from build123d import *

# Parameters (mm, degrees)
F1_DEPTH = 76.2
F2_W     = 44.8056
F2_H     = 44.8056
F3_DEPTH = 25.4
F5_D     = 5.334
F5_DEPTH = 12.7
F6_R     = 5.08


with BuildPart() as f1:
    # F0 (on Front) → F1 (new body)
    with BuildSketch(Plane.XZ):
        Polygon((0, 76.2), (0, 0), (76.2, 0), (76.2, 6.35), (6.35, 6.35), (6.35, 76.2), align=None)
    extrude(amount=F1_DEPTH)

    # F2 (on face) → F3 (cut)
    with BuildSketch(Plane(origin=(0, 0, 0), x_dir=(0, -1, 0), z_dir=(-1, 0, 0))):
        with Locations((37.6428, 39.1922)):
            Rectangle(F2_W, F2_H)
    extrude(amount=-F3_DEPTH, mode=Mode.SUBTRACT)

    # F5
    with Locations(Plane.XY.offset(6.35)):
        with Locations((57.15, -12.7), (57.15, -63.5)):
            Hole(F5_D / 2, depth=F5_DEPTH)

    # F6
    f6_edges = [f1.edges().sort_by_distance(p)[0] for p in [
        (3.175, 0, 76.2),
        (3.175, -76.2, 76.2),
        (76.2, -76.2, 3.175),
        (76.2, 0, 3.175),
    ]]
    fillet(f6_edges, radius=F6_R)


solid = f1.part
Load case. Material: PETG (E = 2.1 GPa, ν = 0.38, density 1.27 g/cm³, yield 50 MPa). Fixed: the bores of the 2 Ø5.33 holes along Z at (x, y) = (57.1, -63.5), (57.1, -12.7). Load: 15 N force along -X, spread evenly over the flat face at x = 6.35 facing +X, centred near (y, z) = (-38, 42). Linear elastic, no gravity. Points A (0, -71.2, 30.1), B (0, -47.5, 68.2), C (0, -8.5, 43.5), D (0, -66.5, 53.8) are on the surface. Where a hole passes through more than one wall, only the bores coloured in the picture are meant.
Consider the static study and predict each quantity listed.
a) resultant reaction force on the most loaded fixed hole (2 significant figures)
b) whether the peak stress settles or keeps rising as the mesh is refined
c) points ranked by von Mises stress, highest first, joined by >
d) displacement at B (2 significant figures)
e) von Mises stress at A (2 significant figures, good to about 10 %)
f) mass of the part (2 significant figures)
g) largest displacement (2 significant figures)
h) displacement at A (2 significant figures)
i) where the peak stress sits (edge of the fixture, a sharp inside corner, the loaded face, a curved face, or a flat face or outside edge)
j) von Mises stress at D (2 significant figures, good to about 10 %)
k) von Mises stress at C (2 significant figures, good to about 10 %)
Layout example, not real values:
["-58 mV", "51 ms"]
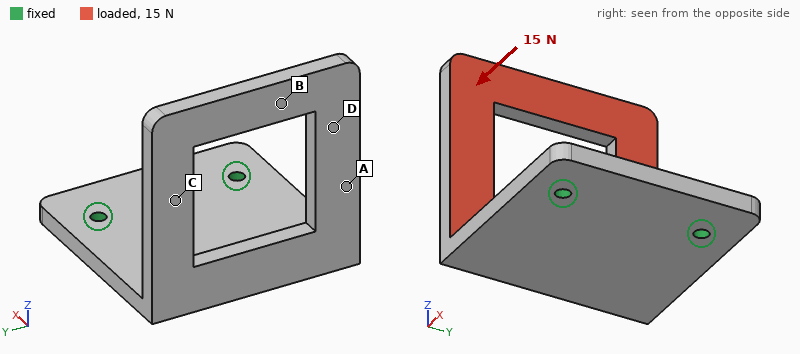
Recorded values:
["7.7 N", "keeps rising", "A > C > D > B", "1.1 mm", "1.3 MPa", "73 g", "1.2 mm", "0.46 mm", "edge of the fixture", "0.41 MPa", "0.74 MPa"]
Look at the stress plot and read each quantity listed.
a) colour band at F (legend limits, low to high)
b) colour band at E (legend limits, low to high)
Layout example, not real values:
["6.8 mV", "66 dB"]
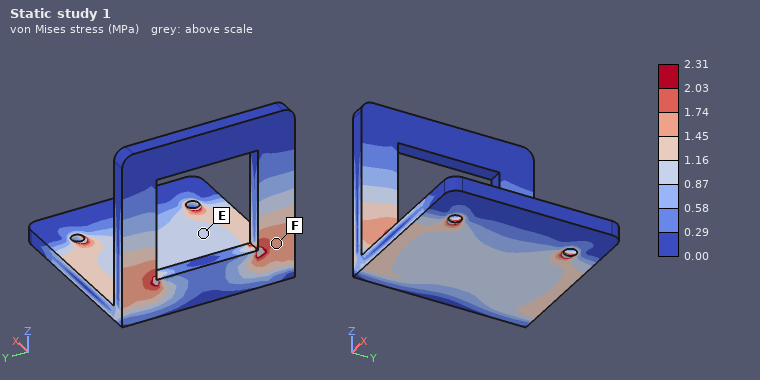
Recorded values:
["1.45 to 1.74 MPa", "0.87 to 1.16 MPa"]
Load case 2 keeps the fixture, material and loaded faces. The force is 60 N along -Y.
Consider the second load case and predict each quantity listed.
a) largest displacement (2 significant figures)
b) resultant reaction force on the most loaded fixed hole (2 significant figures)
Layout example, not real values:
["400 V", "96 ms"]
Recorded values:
["1.4 mm", "78 N"]
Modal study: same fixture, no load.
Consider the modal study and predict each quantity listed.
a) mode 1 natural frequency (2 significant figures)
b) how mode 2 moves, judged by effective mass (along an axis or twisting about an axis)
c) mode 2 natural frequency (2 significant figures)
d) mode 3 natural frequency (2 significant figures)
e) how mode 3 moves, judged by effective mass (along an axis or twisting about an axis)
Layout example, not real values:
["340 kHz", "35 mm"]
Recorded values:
["120 Hz", "along Y", "220 Hz", "290 Hz", "along Z"]
